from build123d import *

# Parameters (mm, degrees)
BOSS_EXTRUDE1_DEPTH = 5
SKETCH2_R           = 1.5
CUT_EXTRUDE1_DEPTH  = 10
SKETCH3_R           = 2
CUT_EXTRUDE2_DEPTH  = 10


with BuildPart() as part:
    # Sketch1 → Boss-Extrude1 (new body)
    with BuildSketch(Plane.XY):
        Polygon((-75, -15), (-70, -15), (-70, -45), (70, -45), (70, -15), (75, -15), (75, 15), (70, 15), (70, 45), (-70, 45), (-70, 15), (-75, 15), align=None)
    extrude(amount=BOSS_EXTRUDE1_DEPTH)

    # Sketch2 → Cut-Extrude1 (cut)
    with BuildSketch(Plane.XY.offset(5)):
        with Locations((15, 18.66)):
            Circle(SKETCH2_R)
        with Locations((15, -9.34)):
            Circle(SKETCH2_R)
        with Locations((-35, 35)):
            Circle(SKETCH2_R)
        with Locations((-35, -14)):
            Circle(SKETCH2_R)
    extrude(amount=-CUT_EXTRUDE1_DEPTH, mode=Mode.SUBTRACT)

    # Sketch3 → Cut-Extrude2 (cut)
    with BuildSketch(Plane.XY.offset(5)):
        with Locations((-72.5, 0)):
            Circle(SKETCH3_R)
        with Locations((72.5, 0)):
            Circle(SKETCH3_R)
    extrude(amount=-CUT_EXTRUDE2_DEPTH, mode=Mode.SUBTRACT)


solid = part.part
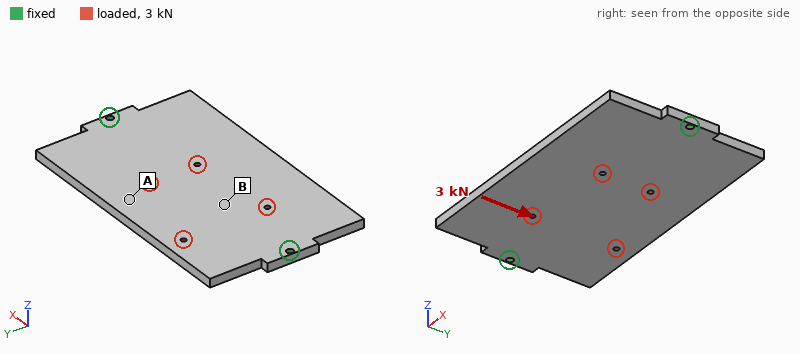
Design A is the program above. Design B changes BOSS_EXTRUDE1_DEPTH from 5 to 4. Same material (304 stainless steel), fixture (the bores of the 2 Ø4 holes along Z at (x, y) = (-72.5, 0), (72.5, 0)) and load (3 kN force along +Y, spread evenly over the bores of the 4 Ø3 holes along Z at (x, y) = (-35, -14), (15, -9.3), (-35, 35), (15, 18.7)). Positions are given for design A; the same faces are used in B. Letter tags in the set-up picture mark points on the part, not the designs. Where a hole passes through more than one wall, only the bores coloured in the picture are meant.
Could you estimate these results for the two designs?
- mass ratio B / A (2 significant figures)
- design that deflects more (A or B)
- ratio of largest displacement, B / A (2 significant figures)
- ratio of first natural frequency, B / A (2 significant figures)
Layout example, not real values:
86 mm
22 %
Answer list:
0.80
B
1.3
0.81
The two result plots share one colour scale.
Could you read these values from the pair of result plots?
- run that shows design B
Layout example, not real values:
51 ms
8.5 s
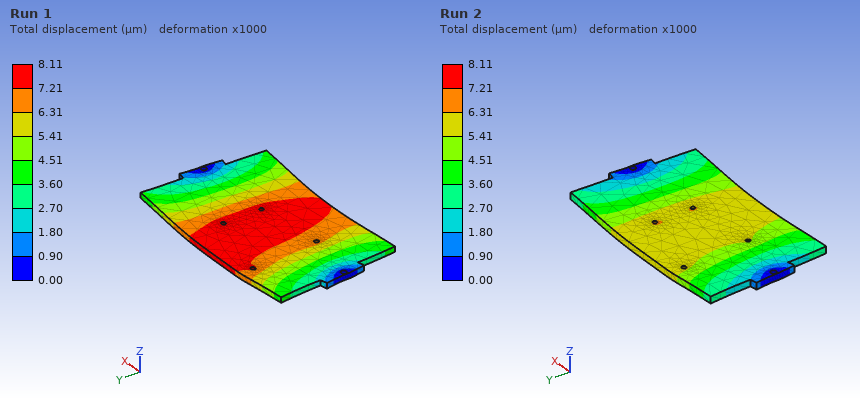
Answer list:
Run 1
